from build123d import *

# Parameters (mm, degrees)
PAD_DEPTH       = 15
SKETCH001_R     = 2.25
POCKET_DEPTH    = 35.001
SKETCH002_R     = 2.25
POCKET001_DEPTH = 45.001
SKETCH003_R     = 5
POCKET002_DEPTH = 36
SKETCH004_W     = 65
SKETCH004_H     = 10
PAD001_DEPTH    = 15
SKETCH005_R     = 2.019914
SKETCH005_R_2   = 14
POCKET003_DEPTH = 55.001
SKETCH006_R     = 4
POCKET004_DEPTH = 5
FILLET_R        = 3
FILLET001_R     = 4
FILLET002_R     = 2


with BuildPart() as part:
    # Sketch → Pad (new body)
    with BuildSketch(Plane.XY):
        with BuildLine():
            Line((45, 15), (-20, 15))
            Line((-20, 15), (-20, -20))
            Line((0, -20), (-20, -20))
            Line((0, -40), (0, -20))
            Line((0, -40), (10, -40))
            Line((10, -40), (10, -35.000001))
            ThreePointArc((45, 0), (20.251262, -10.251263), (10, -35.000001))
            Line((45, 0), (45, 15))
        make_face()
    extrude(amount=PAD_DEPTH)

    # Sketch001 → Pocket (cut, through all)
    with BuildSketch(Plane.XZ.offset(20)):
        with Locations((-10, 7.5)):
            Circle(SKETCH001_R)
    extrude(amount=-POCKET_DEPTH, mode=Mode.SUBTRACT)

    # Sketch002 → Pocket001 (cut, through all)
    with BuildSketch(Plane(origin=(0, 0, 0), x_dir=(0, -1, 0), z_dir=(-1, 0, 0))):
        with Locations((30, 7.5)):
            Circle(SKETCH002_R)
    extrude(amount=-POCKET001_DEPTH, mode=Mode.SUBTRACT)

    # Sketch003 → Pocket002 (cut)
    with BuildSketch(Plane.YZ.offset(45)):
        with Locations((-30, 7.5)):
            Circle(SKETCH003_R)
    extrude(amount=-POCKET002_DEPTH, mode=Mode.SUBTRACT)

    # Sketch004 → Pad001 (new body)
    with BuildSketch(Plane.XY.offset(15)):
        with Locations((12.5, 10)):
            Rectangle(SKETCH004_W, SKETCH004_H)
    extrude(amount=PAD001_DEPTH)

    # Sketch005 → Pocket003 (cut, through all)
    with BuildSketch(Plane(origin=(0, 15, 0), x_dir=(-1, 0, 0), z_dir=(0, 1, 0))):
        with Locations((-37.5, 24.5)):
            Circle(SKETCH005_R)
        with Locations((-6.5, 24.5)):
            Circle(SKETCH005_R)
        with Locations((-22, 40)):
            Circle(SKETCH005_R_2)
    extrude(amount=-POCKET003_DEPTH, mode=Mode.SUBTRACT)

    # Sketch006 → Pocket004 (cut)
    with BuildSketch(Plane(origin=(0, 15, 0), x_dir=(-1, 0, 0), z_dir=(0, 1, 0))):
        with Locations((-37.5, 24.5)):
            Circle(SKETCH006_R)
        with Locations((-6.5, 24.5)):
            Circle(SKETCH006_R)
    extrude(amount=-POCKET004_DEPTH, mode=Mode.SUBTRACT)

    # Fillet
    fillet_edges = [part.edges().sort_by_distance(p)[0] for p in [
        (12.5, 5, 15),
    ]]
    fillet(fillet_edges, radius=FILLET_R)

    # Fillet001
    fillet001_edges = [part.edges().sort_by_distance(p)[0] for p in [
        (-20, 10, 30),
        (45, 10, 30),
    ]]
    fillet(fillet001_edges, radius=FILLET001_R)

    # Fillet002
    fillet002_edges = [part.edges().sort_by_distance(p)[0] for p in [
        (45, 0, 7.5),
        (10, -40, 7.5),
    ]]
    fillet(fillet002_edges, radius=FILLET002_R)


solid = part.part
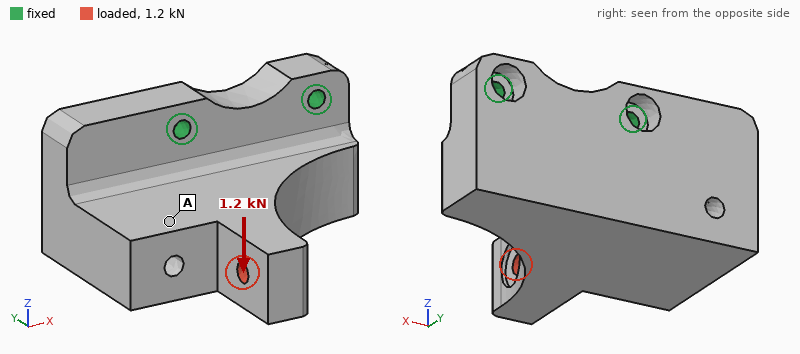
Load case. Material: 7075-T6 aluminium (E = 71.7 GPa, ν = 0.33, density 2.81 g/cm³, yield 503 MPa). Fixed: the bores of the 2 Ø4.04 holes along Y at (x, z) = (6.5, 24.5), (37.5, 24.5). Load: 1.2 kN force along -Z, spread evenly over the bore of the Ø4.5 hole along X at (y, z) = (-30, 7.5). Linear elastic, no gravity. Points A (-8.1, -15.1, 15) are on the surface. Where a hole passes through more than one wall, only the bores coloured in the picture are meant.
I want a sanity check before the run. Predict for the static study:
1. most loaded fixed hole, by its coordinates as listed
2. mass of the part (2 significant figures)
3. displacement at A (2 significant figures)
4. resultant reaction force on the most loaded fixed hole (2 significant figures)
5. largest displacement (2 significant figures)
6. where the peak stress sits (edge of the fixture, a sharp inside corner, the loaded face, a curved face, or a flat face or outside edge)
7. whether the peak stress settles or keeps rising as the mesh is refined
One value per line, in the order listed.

(6.5, 24.5)
110 g
0.16 mm
1.3 kN
0.37 mm
edge of the fixture
keeps rising
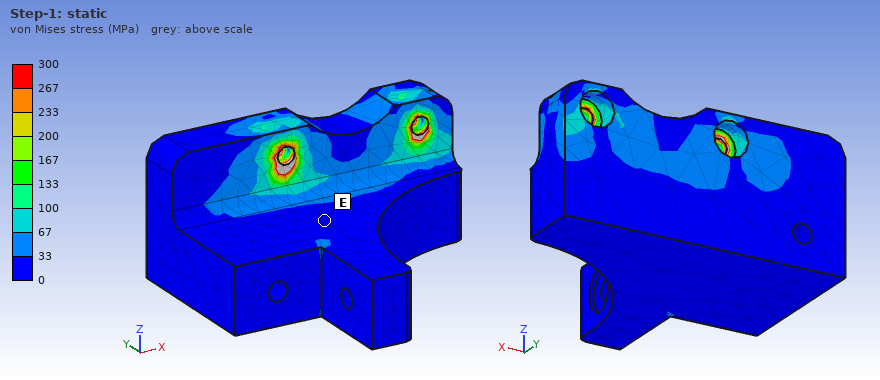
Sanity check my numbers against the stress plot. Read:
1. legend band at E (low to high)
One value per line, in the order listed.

0 to 33 MPa
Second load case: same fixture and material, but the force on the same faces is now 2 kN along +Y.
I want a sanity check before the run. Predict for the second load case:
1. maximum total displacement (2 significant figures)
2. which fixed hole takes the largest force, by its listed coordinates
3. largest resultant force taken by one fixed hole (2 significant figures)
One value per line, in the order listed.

0.22 mm
(6.5, 24.5)
2.0 kN
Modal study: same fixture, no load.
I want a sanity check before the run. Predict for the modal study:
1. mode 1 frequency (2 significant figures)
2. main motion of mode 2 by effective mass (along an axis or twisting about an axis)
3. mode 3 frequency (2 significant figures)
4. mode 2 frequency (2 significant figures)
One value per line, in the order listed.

2000 Hz
along X
8100 Hz
4500 Hz
